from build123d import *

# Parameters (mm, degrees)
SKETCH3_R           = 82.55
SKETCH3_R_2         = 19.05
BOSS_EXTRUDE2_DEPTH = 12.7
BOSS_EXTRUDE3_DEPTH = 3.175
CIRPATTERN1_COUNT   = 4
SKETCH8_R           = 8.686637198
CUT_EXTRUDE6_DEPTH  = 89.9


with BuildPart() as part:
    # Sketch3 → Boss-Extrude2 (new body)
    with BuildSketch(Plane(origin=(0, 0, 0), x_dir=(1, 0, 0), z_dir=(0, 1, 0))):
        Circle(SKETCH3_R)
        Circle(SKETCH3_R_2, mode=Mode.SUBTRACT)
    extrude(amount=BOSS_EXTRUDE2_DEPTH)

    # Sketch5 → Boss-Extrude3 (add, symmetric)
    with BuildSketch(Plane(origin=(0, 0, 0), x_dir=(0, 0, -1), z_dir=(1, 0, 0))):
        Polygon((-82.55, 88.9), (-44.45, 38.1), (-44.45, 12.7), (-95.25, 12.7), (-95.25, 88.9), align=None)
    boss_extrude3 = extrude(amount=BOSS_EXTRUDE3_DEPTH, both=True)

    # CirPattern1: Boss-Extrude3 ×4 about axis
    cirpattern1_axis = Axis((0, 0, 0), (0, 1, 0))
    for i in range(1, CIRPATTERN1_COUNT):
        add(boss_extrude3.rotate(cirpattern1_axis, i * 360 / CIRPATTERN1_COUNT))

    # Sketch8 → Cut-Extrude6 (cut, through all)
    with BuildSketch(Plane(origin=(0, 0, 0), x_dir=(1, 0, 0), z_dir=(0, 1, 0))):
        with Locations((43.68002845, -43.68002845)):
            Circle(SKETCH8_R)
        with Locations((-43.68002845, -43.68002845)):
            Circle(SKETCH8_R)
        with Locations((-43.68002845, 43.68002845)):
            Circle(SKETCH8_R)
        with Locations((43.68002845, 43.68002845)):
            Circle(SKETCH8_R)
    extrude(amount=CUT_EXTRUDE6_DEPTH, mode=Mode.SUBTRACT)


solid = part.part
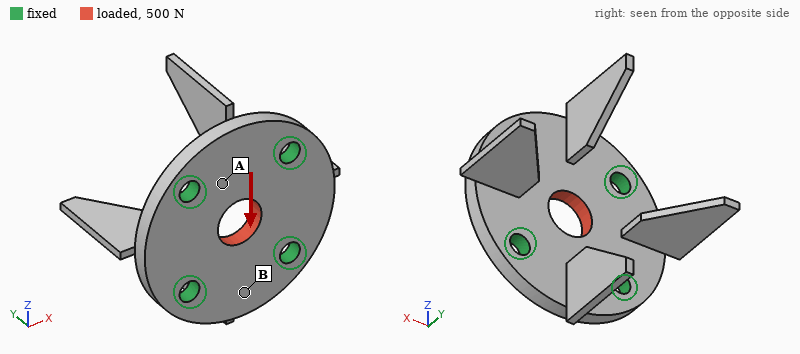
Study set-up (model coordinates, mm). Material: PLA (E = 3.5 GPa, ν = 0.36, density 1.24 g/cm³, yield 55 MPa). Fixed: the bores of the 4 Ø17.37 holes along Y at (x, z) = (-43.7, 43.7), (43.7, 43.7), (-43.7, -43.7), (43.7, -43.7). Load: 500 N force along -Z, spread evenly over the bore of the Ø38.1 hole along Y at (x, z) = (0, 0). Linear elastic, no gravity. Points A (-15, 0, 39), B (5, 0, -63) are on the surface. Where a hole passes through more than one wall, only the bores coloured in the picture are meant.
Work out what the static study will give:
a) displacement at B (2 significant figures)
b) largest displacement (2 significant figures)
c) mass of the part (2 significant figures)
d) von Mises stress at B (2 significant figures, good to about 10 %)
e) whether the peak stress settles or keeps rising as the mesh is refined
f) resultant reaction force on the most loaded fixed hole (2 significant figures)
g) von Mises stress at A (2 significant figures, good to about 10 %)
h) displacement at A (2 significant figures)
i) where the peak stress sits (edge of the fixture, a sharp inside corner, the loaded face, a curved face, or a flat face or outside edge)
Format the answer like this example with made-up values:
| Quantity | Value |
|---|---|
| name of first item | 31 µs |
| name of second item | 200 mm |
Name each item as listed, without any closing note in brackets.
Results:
| Quantity | Value |
|---|---|
| displacement at B | 2.5 µm |
| largest displacement | 4.8 µm |
| mass of the part | 400 g |
| von Mises stress at B | 0.10 MPa |
| whether the peak stress settles or keeps rising as the mesh is refined | keeps rising |
| resultant reaction force on the most loaded fixed hole | 130 N |
| von Mises stress at A | 0.20 MPa |
| displacement at A | 2.7 µm |
| where the peak stress sits | edge of the fixture |
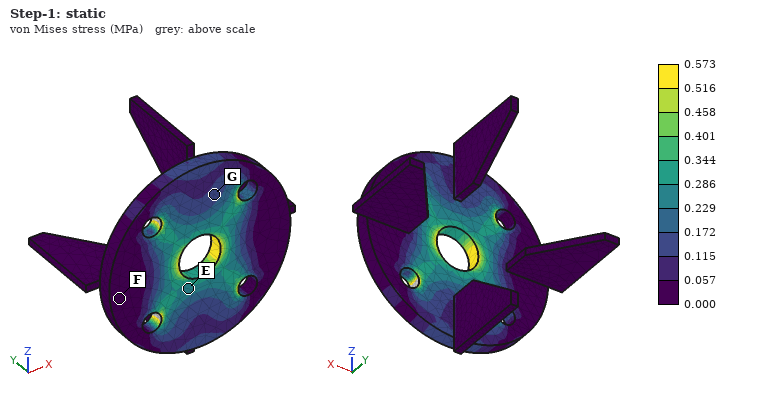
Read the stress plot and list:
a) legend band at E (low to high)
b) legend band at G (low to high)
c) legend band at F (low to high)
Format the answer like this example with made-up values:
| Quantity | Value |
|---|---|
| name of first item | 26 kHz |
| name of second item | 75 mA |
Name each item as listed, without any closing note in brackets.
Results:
| Quantity | Value |
|---|---|
| legend band at E | 0.229 to 0.286 MPa |
| legend band at G | 0.115 to 0.172 MPa |
| legend band at F | 0.000 to 0.057 MPa |
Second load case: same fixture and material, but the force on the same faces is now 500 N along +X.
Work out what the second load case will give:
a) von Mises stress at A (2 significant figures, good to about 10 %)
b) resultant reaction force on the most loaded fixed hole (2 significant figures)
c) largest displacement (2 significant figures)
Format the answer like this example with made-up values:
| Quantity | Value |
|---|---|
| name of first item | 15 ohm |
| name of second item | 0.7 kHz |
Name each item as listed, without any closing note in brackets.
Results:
| Quantity | Value |
|---|---|
| von Mises stress at A | 0.16 MPa |
| resultant reaction force on the most loaded fixed hole | 130 N |
| largest displacement | 4.8 µm |
